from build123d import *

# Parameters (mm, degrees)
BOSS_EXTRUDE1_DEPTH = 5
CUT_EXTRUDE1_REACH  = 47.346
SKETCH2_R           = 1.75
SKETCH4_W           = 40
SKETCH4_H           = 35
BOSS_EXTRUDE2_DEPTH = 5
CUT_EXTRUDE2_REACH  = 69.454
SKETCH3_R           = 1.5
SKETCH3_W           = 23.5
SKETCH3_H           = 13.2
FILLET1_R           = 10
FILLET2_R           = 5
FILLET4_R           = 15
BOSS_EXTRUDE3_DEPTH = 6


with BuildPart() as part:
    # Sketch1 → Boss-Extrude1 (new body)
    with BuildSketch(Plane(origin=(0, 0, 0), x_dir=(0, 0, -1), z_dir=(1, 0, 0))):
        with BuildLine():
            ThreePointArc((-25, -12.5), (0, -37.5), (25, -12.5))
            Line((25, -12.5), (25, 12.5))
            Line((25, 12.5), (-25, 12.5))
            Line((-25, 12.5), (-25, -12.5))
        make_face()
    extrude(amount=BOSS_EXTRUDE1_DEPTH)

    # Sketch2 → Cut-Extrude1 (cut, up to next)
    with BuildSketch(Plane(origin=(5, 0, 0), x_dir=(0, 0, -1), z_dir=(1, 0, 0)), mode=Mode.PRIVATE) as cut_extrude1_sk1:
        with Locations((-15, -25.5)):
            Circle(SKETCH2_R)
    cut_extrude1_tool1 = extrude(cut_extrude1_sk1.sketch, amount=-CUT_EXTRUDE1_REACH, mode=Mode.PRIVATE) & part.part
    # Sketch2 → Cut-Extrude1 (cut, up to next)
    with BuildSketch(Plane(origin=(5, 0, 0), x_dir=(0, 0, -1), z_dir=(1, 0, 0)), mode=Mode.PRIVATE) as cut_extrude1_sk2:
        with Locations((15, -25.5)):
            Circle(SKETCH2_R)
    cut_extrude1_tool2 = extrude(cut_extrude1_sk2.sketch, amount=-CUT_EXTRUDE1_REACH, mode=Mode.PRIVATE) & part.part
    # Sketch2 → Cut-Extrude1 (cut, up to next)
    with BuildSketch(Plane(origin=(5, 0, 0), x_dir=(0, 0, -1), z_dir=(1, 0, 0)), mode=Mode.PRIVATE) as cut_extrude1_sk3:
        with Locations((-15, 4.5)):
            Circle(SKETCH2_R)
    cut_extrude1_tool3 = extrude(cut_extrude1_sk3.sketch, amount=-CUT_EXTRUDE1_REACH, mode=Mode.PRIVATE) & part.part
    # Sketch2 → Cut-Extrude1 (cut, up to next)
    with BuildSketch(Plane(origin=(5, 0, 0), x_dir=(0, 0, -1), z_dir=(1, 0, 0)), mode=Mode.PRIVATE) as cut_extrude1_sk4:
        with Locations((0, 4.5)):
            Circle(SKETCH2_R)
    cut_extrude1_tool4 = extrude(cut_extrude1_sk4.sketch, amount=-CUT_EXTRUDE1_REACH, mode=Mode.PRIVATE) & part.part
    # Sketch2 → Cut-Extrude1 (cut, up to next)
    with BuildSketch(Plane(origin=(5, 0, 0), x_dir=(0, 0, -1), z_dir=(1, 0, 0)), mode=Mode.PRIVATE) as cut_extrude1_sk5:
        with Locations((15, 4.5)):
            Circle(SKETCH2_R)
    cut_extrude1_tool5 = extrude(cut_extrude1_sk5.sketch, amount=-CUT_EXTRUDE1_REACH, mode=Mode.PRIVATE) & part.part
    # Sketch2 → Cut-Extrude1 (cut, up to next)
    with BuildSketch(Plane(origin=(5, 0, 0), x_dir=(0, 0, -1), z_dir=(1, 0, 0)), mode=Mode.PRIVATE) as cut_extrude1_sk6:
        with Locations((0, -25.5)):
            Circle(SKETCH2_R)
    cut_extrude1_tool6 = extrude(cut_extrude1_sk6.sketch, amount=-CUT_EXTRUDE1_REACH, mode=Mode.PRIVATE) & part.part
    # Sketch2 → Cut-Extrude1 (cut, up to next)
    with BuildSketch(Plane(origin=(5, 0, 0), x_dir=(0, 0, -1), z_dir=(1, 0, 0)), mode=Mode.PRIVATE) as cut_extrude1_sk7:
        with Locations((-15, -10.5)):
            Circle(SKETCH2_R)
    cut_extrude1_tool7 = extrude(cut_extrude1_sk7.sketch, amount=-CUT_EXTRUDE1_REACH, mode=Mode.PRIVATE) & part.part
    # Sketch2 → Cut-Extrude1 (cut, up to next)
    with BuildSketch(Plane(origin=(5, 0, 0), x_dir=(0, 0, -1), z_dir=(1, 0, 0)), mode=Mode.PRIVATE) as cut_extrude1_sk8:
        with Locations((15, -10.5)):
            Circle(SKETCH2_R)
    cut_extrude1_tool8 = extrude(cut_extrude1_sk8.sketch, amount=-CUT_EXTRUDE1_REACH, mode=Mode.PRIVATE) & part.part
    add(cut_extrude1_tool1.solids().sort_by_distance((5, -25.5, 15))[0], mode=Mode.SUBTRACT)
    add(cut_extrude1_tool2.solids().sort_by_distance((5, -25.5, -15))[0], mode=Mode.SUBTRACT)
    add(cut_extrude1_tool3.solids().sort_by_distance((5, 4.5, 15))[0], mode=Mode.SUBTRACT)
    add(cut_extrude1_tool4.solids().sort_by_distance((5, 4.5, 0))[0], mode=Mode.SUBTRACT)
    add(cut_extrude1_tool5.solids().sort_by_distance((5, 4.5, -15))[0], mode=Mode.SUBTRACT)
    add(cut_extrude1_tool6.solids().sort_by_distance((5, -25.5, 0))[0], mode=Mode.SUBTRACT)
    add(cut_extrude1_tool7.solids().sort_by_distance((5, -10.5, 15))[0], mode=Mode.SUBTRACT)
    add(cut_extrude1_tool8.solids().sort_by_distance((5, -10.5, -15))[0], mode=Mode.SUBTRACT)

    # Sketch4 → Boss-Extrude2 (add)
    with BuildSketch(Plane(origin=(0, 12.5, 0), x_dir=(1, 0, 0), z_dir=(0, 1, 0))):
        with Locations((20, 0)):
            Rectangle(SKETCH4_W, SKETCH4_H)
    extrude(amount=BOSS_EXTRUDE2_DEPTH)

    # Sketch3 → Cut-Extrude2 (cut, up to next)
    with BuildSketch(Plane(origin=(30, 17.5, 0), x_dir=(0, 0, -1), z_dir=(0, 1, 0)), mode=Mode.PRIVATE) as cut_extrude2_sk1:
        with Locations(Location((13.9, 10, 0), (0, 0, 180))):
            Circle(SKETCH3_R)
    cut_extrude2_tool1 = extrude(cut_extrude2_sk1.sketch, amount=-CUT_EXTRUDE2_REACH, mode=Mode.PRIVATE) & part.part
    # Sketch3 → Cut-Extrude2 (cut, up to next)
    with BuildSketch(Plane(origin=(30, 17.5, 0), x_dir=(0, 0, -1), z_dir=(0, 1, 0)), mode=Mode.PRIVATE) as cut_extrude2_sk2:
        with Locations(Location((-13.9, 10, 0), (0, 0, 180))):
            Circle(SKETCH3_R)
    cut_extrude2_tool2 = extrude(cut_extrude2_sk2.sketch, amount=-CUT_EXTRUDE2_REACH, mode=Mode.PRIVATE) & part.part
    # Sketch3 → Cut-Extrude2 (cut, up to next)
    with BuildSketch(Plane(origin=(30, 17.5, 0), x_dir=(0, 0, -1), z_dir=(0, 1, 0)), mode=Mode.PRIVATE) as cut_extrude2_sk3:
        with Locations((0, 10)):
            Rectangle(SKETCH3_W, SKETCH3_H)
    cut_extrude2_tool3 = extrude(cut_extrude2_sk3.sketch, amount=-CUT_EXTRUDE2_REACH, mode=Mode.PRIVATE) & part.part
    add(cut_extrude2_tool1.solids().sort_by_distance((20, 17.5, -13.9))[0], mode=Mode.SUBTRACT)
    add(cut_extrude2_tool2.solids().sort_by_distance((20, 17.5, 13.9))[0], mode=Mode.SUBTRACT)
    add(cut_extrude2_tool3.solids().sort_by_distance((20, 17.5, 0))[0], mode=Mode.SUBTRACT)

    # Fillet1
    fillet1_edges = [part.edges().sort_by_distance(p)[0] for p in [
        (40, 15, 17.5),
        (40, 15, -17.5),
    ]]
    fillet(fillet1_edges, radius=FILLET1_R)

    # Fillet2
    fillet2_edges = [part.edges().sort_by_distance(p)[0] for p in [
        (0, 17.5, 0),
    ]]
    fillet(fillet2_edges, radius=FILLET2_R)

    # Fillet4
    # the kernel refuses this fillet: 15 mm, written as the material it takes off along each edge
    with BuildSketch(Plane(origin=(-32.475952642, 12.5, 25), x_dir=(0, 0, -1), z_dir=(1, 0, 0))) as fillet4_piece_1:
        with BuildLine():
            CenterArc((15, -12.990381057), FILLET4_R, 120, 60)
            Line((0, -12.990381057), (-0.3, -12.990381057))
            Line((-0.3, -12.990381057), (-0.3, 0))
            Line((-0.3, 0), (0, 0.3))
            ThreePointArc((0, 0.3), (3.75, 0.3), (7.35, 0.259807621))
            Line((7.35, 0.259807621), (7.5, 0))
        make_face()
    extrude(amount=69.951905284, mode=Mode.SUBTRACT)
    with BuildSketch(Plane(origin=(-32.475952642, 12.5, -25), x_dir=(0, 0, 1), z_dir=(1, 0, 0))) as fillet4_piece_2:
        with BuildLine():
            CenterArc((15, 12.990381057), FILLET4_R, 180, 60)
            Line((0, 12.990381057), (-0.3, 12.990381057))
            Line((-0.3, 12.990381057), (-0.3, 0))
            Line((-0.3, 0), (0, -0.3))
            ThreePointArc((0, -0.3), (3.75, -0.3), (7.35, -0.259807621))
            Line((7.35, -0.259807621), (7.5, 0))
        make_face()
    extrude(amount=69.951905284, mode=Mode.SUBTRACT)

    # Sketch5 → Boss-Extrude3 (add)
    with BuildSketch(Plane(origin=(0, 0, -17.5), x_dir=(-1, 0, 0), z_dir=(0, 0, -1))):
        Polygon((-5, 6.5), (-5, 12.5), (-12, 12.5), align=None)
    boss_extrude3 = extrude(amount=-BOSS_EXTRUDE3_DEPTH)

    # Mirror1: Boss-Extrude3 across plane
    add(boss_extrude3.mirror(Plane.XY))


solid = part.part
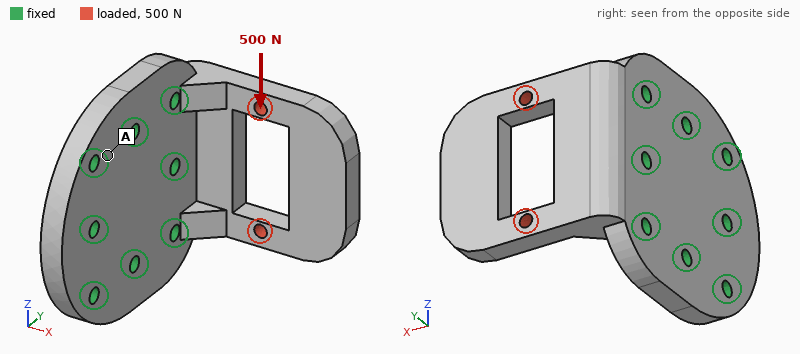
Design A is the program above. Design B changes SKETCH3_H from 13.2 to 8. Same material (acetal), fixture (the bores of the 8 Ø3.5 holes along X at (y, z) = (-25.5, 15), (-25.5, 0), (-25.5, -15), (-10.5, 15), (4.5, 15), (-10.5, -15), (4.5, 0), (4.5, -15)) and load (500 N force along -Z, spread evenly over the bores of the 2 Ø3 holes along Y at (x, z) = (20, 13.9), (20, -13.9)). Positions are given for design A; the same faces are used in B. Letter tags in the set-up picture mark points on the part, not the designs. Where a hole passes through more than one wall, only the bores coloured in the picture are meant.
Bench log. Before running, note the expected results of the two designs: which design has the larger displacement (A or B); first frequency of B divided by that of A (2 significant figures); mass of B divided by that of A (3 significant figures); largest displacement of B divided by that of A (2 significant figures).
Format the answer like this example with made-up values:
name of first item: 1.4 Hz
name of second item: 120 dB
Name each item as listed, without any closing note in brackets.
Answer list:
which design has the larger displacement: A
first frequency of B divided by that of A: 1.0
mass of B divided by that of A: 1.04
largest displacement of B divided by that of A: 0.75
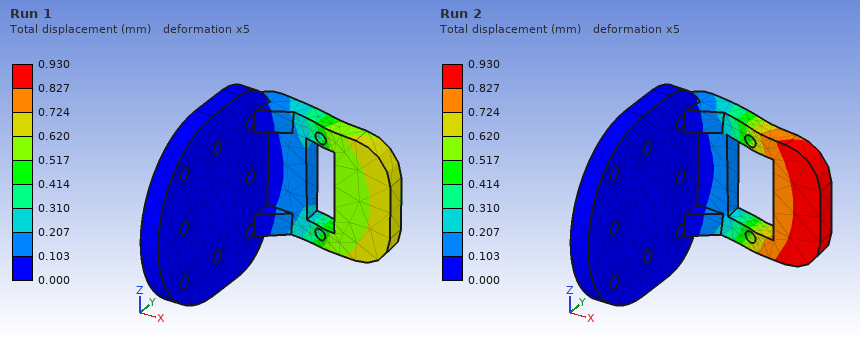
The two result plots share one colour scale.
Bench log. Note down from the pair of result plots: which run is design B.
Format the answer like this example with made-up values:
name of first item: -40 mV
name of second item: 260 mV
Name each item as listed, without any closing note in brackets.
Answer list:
which run is design B: Run 1
